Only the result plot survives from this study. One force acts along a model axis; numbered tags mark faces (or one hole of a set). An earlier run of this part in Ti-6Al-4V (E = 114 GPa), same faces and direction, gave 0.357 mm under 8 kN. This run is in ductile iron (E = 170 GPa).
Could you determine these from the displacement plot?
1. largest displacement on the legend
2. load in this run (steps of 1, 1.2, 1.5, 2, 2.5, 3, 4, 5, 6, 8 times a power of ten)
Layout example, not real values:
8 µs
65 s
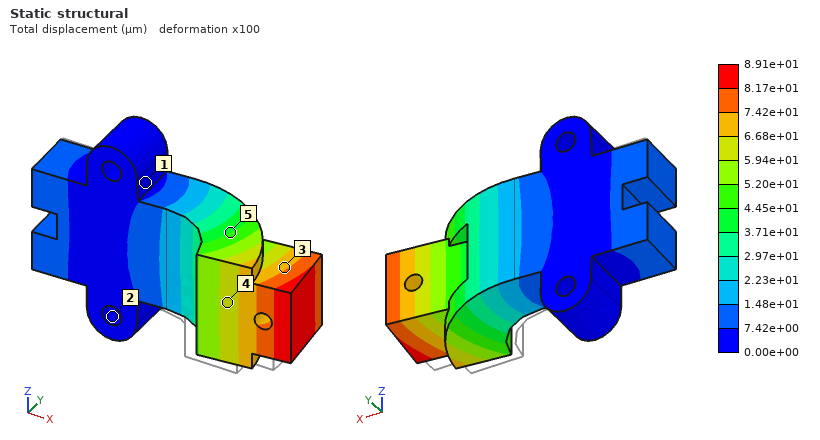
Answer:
8.91e+01 µm
3 kN
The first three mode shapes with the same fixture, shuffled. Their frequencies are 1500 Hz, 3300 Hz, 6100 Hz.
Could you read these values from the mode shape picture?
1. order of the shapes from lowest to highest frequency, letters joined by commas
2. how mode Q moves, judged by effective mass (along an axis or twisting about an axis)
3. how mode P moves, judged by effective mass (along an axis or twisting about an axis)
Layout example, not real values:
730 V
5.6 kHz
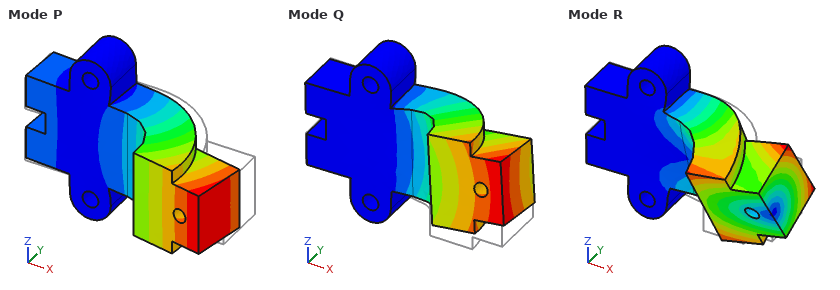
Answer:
P, Q, R
along Z
along Y
